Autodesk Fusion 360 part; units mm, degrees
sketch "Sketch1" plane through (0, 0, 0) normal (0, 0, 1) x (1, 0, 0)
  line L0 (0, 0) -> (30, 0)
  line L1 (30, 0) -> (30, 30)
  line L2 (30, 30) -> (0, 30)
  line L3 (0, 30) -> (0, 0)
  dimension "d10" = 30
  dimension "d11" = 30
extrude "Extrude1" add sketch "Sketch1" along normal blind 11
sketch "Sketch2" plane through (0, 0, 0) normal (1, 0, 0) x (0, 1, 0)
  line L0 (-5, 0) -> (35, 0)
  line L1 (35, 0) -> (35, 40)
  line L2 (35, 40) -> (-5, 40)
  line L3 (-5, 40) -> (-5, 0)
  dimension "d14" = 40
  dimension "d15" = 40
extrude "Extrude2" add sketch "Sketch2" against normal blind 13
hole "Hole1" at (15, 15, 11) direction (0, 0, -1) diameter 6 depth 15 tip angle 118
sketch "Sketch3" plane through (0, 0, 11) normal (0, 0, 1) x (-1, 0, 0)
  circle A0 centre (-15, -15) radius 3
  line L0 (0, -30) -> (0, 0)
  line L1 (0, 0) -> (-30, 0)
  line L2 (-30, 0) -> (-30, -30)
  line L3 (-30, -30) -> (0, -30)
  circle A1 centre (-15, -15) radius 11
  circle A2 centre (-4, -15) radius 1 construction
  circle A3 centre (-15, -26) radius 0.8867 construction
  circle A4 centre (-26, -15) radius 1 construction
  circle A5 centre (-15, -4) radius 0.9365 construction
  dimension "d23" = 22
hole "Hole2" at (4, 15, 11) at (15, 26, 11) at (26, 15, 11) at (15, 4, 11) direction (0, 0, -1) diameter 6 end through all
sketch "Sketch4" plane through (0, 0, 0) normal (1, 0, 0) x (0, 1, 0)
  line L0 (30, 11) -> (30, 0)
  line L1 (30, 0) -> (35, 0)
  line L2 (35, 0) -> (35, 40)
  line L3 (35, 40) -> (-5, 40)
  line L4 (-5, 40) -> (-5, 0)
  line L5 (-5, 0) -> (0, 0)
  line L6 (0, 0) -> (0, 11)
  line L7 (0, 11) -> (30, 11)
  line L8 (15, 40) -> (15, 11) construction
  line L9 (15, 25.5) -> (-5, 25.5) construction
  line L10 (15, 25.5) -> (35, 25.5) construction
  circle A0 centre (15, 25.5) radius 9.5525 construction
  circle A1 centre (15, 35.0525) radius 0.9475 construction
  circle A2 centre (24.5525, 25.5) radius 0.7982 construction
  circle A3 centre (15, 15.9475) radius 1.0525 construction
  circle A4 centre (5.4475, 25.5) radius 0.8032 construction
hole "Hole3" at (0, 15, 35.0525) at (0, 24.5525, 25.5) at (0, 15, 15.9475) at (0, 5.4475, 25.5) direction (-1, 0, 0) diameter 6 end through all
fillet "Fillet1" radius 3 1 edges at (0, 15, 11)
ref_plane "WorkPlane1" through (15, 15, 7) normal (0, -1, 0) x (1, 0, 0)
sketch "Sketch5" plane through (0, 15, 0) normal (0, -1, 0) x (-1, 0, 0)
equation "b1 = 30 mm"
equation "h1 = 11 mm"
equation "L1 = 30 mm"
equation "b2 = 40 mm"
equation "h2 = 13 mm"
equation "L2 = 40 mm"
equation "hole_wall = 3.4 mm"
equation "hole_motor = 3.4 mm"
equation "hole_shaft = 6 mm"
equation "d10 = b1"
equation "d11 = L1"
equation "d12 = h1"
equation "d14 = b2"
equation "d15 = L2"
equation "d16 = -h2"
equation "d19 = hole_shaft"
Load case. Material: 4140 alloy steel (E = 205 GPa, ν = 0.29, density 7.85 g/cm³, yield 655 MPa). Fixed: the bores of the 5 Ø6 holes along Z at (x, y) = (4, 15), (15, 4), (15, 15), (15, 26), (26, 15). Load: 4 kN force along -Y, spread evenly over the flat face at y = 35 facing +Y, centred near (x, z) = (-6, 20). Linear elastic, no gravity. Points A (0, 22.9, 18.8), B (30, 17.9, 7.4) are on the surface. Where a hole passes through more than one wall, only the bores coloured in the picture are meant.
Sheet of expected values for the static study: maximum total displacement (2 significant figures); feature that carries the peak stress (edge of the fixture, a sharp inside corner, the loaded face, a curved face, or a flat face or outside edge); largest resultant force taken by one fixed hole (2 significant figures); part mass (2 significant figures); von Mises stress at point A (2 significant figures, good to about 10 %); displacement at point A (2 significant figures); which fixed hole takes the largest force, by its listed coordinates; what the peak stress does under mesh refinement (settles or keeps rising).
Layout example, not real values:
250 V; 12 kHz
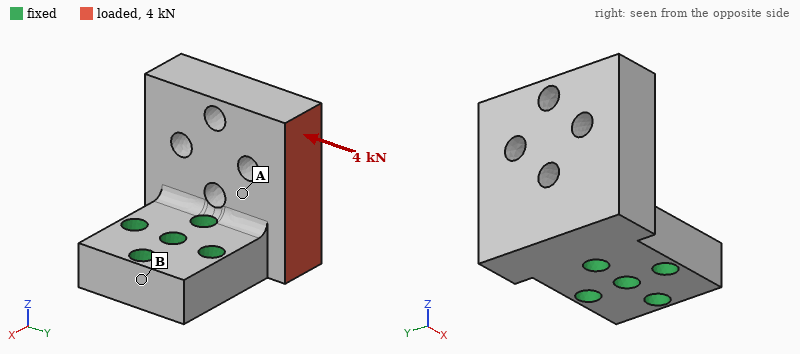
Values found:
22 µm; edge of the fixture; 4.2 kN; 220 g; 24 MPa; 8.7 µm; (4, 15); keeps rising
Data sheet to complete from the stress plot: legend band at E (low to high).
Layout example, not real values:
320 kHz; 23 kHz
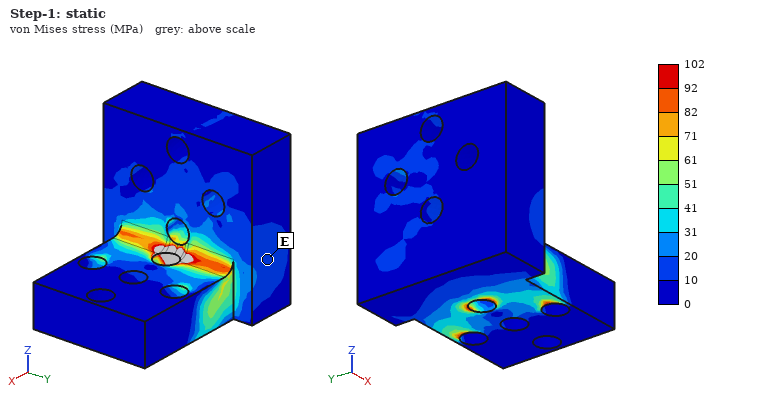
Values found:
10 to 20 MPa
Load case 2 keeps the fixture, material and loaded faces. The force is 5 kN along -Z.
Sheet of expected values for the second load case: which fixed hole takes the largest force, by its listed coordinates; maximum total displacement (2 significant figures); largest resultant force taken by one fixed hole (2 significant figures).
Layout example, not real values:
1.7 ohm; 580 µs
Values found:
(4, 15); 46 µm; 5.0 kN
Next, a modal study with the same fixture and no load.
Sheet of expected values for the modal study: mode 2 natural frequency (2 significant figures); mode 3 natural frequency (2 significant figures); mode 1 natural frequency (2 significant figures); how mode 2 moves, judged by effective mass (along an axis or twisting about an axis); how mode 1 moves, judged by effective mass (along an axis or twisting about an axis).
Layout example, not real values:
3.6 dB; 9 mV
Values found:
6300 Hz; 11 kHz; 5200 Hz; along Y; along X
